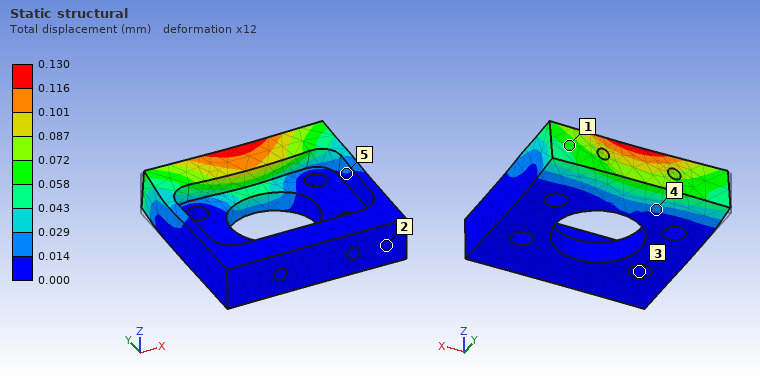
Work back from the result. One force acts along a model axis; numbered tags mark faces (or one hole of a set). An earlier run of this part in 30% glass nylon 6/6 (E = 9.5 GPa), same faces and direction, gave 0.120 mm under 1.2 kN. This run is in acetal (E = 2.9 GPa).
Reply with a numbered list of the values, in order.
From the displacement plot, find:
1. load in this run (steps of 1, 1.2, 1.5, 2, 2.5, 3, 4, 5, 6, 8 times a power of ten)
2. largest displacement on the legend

1. 400 N
2. 0.130 mm
